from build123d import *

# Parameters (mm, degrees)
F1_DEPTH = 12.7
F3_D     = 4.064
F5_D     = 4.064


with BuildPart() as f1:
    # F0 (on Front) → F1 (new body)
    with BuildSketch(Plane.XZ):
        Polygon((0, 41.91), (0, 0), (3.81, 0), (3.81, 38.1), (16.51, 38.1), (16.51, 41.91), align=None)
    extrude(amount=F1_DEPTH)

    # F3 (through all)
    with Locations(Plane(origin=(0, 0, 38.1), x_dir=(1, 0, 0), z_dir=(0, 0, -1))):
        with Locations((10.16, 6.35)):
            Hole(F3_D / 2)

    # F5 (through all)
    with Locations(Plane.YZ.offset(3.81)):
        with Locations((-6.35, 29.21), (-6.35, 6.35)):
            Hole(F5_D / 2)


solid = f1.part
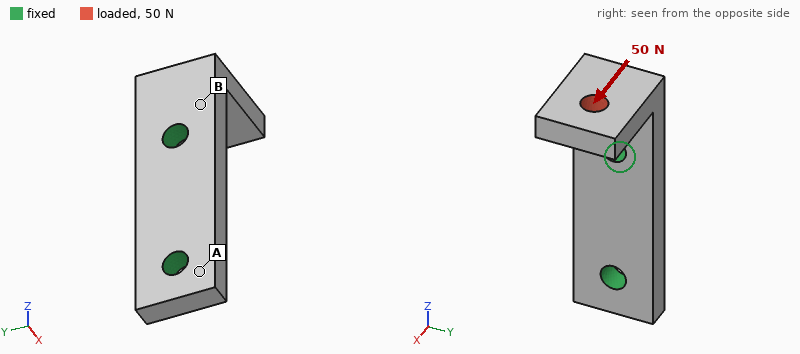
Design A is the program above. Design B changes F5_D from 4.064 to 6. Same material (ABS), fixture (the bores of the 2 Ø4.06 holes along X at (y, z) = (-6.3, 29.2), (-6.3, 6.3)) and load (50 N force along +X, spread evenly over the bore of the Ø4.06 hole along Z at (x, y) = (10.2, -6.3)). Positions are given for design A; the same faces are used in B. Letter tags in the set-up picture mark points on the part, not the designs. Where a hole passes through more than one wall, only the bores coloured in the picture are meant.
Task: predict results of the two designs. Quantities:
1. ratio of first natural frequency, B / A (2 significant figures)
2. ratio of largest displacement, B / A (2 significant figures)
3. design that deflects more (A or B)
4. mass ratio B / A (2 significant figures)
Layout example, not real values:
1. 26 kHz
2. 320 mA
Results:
1. 1.1
2. 0.76
3. A
4. 0.95
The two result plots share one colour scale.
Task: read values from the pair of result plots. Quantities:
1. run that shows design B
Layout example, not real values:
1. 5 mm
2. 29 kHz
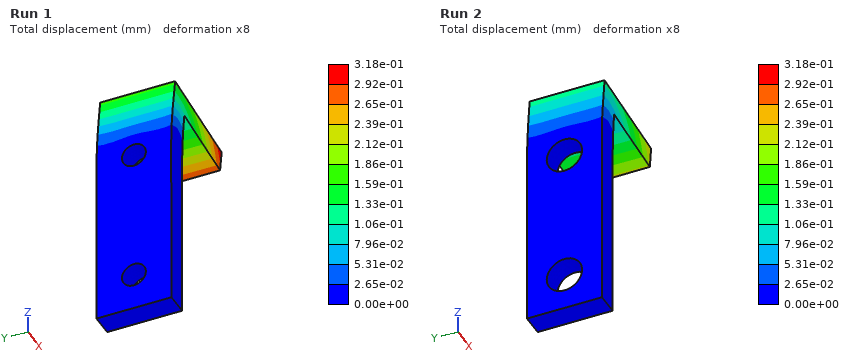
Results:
1. Run 2
